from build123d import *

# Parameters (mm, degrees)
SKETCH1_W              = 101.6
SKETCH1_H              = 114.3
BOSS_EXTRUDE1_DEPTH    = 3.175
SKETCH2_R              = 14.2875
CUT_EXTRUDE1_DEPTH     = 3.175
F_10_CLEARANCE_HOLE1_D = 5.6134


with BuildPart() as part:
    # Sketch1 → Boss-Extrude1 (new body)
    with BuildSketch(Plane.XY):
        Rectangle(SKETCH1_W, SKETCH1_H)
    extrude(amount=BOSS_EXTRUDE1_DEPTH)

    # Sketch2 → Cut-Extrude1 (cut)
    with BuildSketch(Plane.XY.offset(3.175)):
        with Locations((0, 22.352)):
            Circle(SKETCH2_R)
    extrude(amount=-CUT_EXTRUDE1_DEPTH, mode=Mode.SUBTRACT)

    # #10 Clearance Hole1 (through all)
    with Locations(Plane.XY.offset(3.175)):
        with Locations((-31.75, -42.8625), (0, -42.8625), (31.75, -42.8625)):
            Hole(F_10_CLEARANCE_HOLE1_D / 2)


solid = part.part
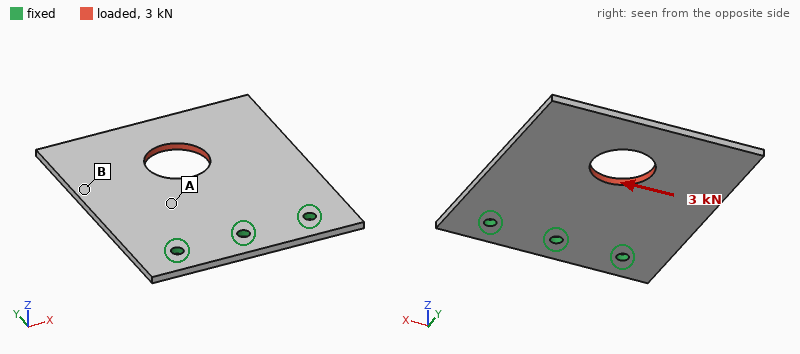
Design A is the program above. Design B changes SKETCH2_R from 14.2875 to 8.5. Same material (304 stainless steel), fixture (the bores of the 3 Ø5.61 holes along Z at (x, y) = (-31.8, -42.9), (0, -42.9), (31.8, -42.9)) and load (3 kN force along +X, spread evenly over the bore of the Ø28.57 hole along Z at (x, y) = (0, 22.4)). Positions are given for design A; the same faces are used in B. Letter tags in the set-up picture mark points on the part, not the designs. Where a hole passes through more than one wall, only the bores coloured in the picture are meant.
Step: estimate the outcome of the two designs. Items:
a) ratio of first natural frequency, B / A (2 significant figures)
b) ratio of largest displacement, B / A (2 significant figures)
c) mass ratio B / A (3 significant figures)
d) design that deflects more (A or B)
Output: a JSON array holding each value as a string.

["0.98", "0.90", "1.04", "A"]
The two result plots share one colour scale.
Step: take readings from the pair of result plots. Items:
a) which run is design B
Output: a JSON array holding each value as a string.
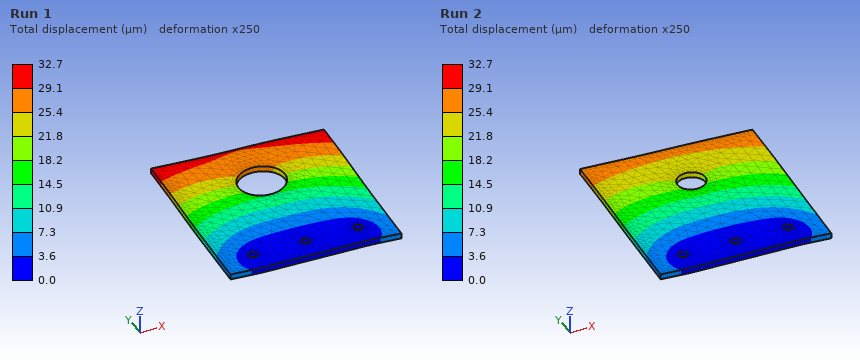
["Run 2"]
